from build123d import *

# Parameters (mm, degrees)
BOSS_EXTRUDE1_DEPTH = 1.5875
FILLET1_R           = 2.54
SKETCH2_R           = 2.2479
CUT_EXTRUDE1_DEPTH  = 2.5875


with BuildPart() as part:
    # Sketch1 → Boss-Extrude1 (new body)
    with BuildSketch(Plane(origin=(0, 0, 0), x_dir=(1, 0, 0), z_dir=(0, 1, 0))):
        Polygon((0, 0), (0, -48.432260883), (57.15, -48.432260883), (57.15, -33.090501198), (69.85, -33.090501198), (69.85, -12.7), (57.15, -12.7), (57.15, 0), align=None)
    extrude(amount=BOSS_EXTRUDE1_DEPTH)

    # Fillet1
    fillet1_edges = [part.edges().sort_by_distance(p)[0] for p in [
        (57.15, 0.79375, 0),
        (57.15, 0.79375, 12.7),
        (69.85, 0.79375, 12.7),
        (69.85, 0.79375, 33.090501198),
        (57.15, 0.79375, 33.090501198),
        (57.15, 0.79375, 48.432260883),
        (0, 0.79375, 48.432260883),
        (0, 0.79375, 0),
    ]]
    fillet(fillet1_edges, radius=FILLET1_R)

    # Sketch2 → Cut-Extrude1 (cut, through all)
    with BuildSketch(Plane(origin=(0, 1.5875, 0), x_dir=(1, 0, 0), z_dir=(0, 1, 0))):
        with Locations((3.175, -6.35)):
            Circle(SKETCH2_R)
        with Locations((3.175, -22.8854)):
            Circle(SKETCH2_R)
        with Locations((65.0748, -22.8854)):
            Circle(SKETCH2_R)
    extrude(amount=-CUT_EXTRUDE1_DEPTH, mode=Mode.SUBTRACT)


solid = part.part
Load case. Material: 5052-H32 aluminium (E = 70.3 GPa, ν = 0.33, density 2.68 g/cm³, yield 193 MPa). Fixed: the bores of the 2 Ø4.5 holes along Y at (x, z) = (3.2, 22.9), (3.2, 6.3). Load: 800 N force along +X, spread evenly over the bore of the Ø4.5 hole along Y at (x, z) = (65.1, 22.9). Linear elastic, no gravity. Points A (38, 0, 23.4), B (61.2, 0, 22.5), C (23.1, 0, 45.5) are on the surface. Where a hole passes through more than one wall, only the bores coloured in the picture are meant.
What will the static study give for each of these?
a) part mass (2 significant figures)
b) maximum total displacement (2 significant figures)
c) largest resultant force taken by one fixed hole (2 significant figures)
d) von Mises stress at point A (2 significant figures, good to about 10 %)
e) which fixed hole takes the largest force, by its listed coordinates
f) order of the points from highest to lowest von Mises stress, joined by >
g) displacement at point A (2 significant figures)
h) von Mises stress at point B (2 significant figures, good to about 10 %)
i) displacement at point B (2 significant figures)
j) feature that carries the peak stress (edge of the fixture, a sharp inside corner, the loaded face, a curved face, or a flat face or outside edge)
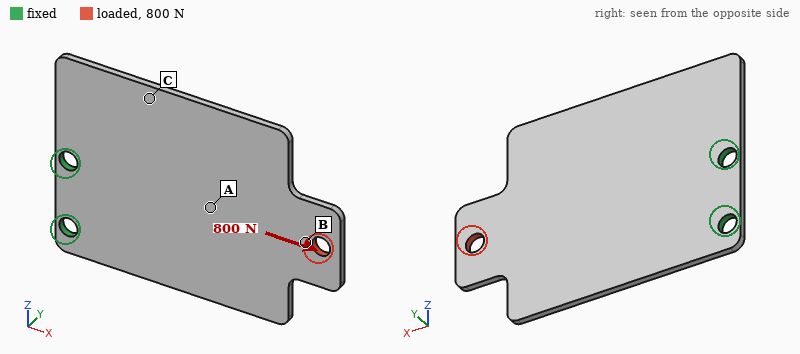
13 g
36 µm
730 N
18 MPa
(3.2, 22.9)
B > A > C
18 µm
36 MPa
29 µm
edge of the fixture
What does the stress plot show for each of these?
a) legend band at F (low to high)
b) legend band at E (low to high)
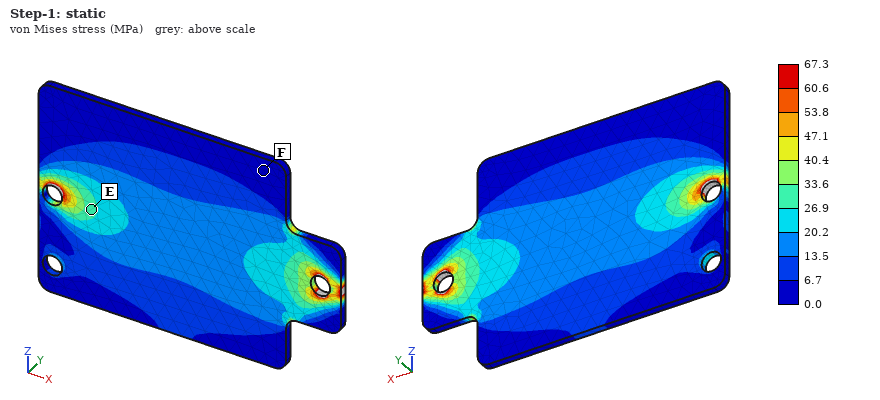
0.0 to 6.7 MPa
26.9 to 33.6 MPa
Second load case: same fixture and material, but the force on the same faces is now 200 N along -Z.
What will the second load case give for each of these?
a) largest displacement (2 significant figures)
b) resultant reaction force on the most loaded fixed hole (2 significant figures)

70 µm
640 N
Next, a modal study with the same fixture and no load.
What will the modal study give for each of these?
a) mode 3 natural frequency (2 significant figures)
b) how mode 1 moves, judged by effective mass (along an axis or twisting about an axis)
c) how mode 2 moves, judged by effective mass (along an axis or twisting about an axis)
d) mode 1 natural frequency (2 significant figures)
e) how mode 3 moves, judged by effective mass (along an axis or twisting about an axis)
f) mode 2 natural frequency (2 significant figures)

1900 Hz
along Y
twisting about X
350 Hz
along Y
980 Hz
